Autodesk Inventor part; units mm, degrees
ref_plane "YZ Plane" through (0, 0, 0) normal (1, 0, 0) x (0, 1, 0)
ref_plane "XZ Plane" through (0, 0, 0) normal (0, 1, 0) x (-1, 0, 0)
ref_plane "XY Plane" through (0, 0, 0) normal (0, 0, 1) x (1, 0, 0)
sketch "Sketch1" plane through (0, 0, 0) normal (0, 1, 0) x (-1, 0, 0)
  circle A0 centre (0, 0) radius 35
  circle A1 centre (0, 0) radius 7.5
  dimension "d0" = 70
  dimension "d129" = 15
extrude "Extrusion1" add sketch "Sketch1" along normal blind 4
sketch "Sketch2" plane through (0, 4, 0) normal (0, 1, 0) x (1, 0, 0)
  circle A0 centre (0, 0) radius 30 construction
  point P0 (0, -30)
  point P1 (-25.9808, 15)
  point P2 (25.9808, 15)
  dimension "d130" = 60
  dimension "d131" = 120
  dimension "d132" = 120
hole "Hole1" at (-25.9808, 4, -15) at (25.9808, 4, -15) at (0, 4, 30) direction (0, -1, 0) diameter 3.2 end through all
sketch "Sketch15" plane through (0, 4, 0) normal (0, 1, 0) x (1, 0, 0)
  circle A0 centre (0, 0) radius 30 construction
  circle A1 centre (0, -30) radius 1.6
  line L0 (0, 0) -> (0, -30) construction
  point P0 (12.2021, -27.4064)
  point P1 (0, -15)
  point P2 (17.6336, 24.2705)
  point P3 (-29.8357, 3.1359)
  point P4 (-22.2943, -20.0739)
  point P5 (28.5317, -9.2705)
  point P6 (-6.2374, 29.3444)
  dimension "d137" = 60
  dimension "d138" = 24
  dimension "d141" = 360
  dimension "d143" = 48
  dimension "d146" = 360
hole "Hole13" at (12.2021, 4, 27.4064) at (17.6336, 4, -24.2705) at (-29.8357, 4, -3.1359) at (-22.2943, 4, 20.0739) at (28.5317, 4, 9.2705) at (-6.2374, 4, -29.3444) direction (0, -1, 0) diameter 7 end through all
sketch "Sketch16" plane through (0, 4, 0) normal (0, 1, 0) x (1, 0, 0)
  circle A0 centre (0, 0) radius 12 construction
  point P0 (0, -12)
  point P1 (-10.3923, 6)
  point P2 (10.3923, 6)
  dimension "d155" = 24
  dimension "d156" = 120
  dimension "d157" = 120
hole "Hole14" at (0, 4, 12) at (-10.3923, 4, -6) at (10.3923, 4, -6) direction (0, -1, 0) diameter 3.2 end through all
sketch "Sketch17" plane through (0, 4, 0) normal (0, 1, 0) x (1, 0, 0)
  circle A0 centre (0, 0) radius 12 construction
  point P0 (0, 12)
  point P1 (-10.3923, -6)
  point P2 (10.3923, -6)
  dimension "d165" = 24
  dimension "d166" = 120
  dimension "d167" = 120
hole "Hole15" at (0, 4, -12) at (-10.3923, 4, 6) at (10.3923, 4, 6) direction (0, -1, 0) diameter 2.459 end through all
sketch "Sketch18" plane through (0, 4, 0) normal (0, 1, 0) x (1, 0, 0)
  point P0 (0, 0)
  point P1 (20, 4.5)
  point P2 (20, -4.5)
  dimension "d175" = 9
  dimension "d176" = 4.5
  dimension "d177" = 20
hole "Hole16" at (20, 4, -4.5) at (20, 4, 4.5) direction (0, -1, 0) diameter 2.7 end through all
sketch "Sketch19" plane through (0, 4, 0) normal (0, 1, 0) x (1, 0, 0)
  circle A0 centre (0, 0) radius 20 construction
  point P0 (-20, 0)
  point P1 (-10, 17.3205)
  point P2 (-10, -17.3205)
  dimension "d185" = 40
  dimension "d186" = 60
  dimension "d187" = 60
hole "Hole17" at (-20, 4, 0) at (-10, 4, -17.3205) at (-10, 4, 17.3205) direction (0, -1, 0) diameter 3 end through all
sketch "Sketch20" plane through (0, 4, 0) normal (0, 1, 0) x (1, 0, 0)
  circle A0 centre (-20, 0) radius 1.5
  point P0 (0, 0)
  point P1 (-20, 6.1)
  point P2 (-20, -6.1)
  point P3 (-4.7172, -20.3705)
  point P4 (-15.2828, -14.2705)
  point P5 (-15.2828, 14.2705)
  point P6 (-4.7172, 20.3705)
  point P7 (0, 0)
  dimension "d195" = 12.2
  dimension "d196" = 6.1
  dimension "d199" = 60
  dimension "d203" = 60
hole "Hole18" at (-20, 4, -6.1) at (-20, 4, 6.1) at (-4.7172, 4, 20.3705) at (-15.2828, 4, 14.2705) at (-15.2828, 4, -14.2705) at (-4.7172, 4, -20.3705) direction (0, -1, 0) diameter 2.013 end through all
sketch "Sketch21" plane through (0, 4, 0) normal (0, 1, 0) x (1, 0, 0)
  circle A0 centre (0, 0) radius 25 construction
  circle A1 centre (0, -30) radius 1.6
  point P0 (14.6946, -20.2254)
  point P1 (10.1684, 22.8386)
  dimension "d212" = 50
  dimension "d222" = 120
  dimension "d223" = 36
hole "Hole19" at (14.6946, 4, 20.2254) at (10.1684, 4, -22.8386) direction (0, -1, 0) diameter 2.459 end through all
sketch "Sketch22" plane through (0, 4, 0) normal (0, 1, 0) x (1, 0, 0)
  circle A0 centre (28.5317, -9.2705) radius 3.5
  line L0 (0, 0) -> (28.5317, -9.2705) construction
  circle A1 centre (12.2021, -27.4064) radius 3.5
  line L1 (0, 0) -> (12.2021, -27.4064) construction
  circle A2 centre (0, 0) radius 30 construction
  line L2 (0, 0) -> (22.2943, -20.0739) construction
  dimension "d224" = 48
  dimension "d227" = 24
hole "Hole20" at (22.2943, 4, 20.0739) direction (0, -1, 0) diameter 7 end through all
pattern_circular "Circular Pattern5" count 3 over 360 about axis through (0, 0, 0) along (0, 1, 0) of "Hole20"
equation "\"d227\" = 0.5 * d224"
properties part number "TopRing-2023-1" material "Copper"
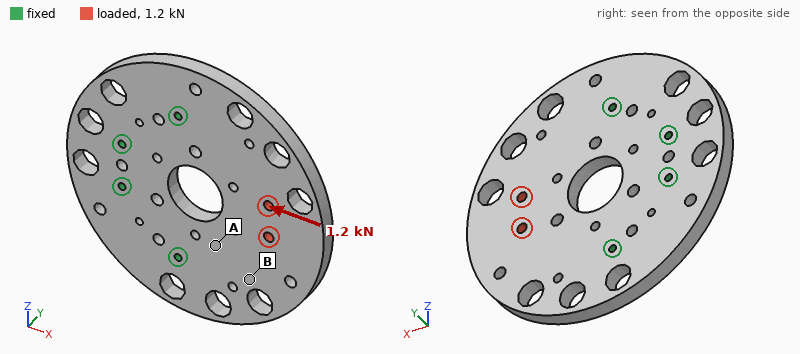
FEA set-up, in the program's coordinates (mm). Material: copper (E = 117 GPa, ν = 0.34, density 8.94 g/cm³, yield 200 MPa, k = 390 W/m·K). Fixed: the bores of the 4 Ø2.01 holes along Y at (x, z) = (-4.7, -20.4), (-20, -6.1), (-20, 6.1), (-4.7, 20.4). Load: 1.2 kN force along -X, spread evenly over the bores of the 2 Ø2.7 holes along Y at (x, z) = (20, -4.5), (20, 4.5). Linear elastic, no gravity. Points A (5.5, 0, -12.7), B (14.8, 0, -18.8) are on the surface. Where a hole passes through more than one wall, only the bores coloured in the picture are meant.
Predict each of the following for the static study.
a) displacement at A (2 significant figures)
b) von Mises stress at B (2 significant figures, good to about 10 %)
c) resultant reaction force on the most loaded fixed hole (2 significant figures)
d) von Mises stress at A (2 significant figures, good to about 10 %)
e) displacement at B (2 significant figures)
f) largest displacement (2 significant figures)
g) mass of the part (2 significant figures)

1.4 µm
4.7 MPa
520 N
9.9 MPa
1.4 µm
4.1 µm
110 g
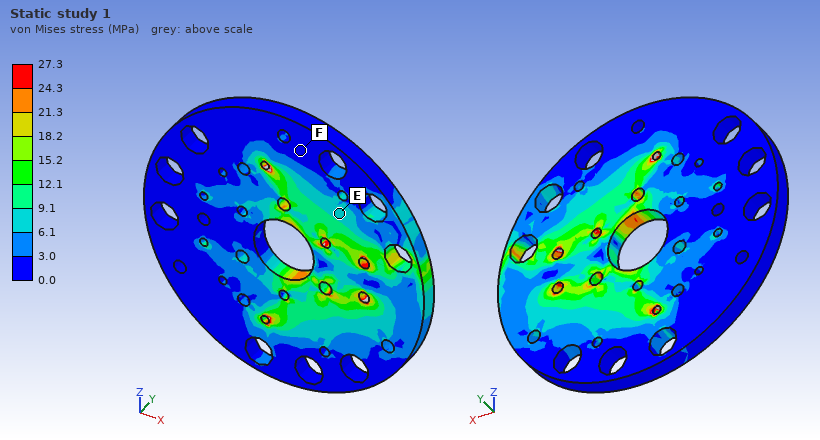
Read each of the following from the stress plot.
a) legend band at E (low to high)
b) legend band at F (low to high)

6.1 to 9.1 MPa
0.0 to 3.0 MPa
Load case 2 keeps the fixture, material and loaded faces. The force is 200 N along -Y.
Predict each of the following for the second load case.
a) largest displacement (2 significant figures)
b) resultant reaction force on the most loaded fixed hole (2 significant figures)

99 µm
140 N
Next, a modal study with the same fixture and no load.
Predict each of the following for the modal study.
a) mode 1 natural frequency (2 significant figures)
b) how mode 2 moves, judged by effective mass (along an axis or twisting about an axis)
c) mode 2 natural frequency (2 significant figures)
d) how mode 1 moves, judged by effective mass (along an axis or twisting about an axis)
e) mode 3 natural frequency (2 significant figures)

1500 Hz
twisting about X
3600 Hz
along Y
6300 Hz
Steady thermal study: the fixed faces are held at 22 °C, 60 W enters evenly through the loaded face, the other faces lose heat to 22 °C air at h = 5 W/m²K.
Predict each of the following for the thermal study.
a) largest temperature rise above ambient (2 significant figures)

34 K
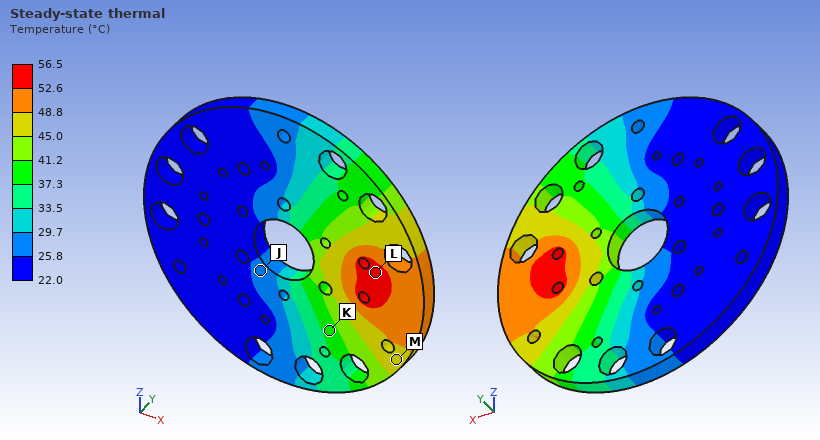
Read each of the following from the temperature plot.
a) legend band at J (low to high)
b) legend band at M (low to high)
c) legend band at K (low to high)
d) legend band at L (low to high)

25.8 to 29.7 °C
45.0 to 48.8 °C
37.3 to 41.2 °C
52.6 to 56.5 °C
